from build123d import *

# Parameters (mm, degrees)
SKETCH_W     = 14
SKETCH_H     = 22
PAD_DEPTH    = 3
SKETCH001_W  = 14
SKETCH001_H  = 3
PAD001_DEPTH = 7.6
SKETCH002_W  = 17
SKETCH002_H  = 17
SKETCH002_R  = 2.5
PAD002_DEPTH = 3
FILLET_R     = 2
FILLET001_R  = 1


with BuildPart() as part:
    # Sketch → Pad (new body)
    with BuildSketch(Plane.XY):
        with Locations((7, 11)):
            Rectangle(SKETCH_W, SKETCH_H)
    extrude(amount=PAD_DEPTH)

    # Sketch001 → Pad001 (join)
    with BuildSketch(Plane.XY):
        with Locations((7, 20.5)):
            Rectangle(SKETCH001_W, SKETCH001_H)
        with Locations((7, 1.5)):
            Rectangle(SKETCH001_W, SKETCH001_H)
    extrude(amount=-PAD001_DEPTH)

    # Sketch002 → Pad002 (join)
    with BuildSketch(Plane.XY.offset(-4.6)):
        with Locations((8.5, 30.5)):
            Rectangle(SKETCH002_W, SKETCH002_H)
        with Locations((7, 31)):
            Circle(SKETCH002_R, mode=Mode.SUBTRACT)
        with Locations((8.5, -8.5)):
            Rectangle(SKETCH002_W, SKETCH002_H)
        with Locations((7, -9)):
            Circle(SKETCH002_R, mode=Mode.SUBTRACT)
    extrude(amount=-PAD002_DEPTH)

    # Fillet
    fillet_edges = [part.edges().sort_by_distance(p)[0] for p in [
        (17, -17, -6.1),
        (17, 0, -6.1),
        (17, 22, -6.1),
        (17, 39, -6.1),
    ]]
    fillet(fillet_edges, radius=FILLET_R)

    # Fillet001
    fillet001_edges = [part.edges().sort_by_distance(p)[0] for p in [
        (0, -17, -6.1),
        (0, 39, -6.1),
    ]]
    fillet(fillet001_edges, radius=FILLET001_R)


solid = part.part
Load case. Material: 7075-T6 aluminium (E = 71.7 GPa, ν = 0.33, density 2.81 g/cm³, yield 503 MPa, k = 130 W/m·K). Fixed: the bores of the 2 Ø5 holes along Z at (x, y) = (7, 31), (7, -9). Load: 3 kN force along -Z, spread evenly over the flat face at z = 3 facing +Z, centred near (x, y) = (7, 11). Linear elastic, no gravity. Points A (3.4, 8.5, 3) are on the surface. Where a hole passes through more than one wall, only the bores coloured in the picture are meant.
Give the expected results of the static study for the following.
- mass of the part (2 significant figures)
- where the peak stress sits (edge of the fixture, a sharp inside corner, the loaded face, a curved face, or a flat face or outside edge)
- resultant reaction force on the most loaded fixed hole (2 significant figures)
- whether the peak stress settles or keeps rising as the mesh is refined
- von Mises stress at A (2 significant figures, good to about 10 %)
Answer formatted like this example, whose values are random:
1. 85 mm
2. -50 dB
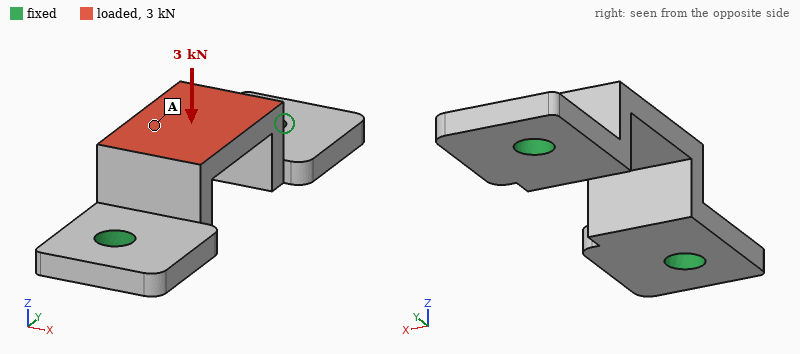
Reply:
1. 8.9 g
2. edge of the fixture
3. 2.0 kN
4. keeps rising
5. 97 MPa
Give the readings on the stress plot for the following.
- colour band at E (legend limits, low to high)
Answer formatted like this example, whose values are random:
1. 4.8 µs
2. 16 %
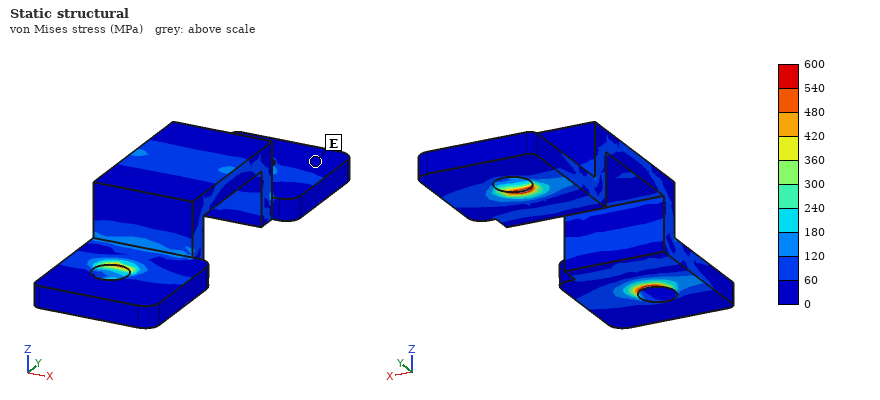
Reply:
1. 0 to 60 MPa
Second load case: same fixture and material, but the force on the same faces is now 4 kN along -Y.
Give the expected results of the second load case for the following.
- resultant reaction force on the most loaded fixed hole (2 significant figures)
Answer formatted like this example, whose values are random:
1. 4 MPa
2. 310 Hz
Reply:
1. 2.3 kN
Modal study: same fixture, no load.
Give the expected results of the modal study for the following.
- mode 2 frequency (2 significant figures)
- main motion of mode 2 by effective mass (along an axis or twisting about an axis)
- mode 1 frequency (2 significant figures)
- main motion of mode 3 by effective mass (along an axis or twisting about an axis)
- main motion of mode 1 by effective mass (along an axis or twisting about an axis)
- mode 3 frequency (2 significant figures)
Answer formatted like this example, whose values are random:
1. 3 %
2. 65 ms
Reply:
1. 15 kHz
2. along Z
3. 9500 Hz
4. along Y
5. along X
6. 16 kHz
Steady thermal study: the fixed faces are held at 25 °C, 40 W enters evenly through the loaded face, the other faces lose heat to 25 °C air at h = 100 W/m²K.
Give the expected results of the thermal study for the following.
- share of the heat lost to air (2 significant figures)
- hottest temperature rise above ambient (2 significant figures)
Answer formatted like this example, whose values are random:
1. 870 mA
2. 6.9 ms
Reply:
1. 13 %
2. 62 K
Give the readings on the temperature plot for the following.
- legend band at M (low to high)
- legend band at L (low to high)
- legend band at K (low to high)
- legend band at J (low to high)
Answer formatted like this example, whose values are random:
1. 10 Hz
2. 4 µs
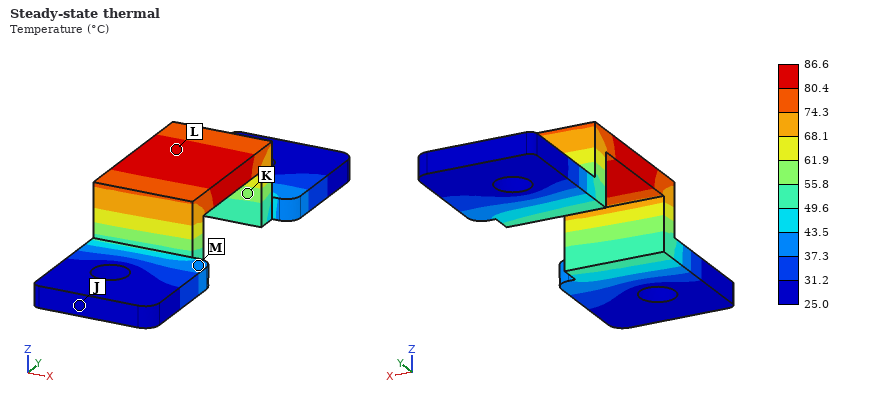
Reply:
1. 37.3 to 43.5 °C
2. 80.4 to 86.6 °C
3. 55.8 to 61.9 °C
4. 25.0 to 31.2 °C
